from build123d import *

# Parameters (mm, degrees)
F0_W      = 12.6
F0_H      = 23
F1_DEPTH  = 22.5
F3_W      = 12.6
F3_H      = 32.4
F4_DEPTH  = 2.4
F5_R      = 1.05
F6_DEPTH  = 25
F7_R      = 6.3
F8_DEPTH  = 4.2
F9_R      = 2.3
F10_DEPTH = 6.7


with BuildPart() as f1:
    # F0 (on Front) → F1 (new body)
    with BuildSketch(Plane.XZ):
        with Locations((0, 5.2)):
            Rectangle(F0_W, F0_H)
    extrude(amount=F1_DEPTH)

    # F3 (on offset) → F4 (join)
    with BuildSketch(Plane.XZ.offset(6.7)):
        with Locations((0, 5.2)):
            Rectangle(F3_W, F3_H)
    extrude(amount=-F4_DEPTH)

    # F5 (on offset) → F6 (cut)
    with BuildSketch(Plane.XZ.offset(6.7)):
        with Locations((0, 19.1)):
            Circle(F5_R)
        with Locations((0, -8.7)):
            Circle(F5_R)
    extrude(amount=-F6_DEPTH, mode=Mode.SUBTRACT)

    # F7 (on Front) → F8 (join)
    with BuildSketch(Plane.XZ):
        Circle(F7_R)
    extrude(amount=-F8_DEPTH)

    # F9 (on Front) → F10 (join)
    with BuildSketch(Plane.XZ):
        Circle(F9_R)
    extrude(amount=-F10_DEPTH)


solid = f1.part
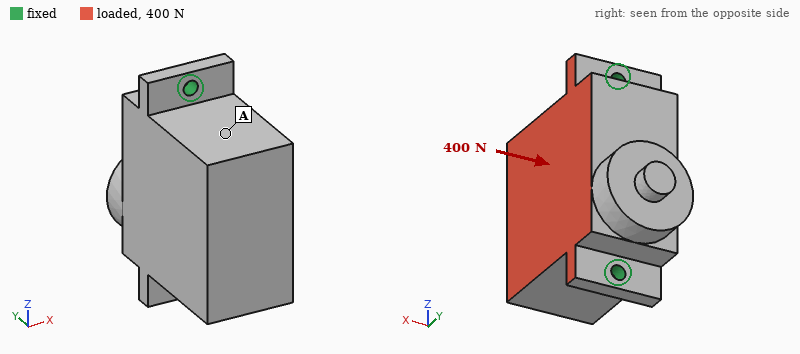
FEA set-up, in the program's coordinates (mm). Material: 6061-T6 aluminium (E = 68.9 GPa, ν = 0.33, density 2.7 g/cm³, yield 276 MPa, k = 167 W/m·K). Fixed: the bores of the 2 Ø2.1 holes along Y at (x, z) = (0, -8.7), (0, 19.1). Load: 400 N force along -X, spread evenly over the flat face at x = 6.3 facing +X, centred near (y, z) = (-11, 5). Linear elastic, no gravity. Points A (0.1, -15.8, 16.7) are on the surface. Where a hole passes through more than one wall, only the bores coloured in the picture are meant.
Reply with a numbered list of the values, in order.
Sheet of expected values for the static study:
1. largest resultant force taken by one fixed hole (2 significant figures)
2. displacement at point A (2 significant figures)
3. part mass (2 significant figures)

1. 200 N
2. 26 µm
3. 20 g
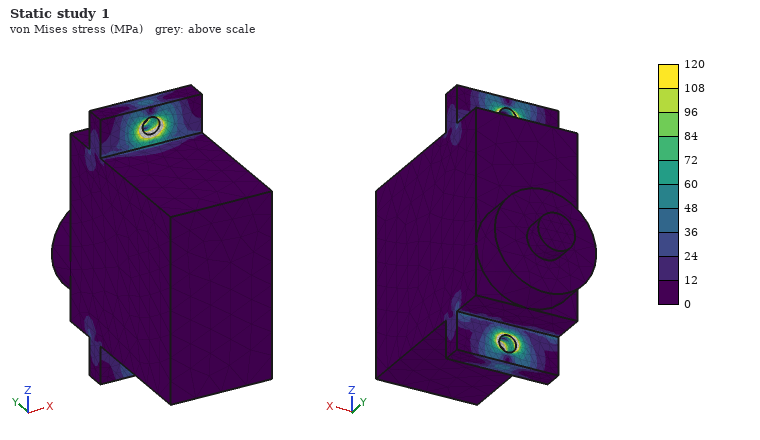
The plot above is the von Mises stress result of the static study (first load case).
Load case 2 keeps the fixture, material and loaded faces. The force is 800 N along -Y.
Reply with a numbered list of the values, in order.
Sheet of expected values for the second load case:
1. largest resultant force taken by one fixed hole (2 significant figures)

1. 400 N
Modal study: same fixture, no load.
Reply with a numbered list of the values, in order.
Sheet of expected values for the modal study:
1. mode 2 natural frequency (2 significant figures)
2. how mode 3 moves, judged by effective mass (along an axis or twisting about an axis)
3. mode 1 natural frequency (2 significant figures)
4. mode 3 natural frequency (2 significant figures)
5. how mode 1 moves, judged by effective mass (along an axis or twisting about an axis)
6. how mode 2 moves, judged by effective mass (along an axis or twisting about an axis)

1. 15 kHz
2. along Z
3. 3700 Hz
4. 16 kHz
5. along X
6. along Y
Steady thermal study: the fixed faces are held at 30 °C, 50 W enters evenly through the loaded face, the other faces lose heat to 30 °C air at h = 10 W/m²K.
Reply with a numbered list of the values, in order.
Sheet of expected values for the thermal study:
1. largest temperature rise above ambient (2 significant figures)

1. 33 K
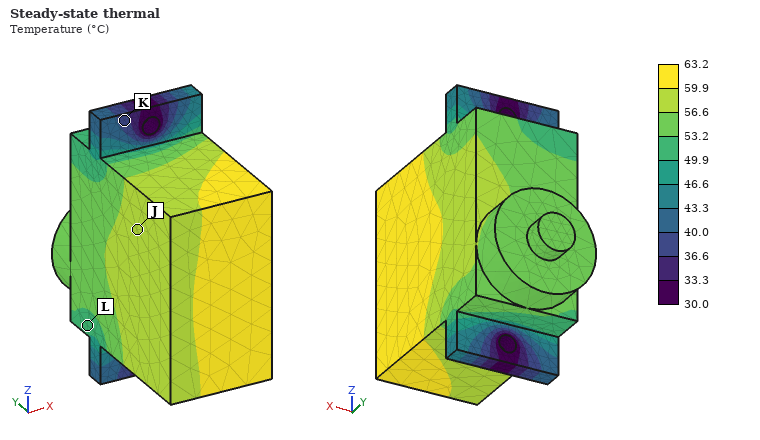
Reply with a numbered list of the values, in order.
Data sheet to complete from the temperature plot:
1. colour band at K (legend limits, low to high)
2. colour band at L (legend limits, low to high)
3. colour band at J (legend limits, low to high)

1. 36.6 to 40.0 °C
2. 49.9 to 53.2 °C
3. 56.6 to 59.9 °C
